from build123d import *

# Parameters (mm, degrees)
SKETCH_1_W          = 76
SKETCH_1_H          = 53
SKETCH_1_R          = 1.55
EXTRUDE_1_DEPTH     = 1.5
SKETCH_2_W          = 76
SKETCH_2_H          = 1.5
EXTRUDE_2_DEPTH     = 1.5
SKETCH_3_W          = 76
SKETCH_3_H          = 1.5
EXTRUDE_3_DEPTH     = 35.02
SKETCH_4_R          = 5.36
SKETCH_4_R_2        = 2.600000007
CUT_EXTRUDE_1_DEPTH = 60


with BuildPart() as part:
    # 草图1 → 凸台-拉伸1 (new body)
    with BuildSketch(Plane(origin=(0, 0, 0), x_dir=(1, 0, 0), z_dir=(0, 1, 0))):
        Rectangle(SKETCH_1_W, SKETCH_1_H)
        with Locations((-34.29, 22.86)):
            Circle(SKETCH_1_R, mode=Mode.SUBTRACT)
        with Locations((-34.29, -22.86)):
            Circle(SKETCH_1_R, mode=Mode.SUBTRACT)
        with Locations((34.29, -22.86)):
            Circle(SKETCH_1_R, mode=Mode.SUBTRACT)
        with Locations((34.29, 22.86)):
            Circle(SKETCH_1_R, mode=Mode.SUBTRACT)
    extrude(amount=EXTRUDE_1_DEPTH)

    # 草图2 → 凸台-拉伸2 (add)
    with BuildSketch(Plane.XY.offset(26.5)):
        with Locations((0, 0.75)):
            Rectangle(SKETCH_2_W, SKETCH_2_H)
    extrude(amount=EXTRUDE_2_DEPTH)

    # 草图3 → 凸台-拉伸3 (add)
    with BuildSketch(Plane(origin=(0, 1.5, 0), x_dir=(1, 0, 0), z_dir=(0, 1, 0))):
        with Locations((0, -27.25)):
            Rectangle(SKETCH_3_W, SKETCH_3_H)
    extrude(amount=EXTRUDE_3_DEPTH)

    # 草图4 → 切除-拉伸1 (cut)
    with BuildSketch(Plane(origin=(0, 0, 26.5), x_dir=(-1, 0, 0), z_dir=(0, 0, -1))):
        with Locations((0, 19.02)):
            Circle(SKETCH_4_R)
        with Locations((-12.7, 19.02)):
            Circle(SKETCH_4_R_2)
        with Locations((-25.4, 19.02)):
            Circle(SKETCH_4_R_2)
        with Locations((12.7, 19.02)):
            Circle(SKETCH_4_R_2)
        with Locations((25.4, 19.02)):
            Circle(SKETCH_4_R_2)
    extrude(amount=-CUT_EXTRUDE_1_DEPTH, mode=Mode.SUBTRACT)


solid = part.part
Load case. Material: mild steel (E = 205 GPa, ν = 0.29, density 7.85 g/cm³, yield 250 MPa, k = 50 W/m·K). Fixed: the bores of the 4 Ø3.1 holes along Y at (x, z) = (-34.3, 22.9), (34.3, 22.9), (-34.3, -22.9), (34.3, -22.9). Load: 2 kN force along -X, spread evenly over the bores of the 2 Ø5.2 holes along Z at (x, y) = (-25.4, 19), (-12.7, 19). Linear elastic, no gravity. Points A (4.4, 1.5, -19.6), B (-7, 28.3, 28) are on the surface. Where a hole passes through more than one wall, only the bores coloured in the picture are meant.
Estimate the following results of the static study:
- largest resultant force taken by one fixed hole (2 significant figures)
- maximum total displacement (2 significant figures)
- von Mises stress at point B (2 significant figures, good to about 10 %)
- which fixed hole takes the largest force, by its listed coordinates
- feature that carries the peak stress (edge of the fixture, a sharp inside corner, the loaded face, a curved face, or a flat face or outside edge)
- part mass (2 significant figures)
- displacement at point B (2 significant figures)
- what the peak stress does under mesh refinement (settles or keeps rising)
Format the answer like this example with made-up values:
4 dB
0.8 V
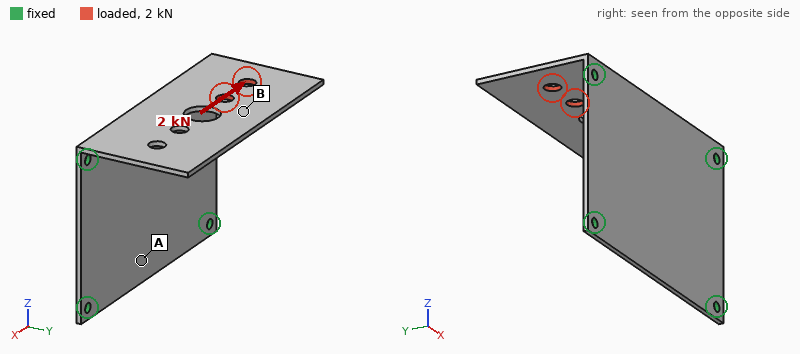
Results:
1.1 kN
81 µm
35 MPa
(-34.3, 22.9)
edge of the fixture
78 g
23 µm
keeps rising
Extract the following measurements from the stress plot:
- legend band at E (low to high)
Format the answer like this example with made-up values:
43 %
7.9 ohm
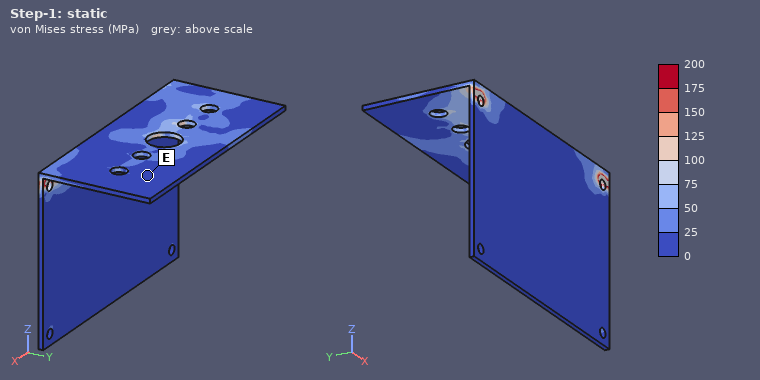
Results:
0 to 25 MPa
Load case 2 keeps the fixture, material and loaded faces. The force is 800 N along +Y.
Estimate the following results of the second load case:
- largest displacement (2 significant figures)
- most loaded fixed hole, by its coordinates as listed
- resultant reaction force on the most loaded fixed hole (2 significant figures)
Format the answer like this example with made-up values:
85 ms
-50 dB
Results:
0.12 mm
(-34.3, 22.9)
660 N
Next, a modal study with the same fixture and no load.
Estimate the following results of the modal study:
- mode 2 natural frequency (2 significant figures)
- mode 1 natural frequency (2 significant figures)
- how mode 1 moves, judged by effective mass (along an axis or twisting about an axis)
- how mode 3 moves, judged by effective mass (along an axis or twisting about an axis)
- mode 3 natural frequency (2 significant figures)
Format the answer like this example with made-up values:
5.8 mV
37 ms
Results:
1300 Hz
730 Hz
along Z
along Y
1700 Hz
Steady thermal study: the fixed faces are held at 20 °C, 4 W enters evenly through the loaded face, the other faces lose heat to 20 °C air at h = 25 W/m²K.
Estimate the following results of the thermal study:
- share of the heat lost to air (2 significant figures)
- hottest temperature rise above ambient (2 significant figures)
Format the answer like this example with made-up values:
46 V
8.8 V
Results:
53 %
27 K
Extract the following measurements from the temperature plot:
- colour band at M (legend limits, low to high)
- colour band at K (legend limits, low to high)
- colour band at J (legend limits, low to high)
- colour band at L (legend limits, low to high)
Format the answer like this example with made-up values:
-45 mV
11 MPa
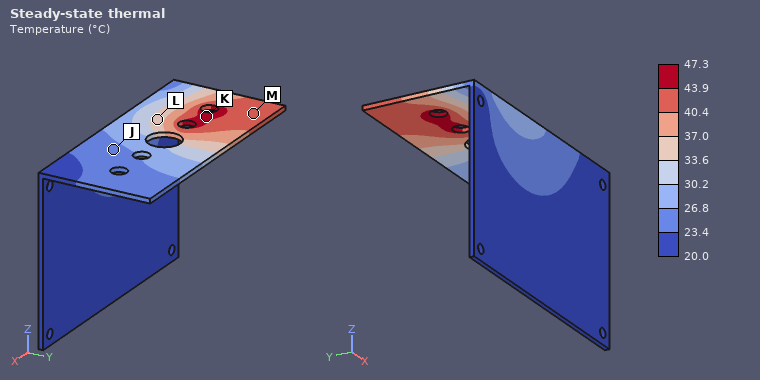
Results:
40.4 to 43.9 °C
43.9 to 47.3 °C
23.4 to 26.8 °C
33.6 to 37.0 °C
